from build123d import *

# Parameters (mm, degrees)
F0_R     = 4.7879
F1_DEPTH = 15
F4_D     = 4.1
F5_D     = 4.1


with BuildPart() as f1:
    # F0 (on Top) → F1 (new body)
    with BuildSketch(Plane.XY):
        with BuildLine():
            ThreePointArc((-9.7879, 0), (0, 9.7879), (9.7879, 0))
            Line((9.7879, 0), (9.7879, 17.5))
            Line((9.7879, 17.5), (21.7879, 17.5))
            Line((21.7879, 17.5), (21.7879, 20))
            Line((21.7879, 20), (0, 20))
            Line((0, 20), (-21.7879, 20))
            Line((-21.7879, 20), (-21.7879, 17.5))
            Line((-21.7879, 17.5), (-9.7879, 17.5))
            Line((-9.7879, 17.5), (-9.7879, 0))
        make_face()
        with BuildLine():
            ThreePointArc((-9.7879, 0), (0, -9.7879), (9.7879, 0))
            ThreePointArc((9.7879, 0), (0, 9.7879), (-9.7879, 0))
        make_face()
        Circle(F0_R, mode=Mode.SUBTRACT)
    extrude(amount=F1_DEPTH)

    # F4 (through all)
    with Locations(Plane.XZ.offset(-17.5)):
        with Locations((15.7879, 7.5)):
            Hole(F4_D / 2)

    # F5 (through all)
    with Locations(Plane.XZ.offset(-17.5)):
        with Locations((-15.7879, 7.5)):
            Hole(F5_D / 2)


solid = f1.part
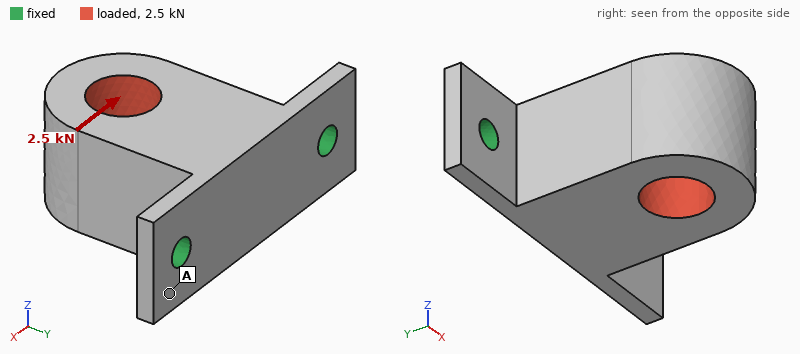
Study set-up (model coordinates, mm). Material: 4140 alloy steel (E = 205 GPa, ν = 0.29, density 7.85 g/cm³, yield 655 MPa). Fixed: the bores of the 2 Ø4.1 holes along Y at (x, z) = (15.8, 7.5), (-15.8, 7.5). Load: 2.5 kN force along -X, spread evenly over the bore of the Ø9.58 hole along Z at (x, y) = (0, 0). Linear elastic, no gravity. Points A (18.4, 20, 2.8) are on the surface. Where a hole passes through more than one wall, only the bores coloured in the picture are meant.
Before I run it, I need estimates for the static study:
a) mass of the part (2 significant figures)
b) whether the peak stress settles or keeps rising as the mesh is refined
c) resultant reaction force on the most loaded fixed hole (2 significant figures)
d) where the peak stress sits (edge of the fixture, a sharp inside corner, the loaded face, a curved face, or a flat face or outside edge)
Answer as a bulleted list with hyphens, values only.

- 62 g
- keeps rising
- 2.3 kN
- edge of the fixture
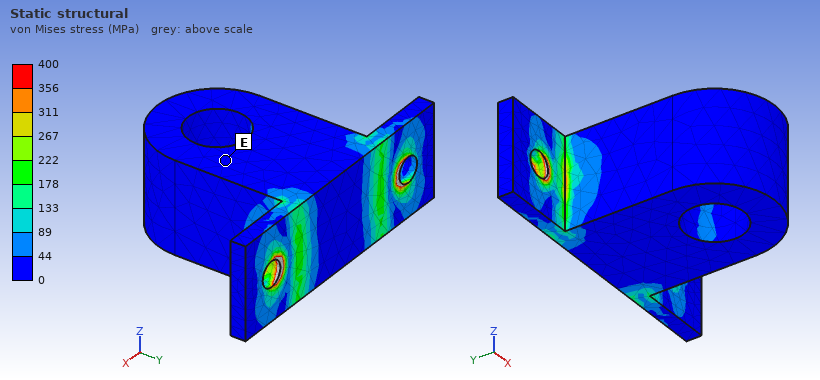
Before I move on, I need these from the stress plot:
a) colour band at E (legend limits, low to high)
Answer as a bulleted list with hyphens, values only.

- 0 to 44 MPa
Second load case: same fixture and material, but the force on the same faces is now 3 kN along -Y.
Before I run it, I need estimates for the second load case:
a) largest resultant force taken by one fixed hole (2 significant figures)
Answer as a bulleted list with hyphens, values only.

- 1.7 kN
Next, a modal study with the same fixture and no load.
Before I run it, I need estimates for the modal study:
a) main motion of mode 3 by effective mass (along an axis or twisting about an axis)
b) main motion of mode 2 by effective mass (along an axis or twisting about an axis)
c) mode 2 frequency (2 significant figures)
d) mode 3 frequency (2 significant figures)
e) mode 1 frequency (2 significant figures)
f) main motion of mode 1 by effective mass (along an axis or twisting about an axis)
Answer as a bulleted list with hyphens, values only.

- along Y
- along X
- 7200 Hz
- 9600 Hz
- 2400 Hz
- along Z
